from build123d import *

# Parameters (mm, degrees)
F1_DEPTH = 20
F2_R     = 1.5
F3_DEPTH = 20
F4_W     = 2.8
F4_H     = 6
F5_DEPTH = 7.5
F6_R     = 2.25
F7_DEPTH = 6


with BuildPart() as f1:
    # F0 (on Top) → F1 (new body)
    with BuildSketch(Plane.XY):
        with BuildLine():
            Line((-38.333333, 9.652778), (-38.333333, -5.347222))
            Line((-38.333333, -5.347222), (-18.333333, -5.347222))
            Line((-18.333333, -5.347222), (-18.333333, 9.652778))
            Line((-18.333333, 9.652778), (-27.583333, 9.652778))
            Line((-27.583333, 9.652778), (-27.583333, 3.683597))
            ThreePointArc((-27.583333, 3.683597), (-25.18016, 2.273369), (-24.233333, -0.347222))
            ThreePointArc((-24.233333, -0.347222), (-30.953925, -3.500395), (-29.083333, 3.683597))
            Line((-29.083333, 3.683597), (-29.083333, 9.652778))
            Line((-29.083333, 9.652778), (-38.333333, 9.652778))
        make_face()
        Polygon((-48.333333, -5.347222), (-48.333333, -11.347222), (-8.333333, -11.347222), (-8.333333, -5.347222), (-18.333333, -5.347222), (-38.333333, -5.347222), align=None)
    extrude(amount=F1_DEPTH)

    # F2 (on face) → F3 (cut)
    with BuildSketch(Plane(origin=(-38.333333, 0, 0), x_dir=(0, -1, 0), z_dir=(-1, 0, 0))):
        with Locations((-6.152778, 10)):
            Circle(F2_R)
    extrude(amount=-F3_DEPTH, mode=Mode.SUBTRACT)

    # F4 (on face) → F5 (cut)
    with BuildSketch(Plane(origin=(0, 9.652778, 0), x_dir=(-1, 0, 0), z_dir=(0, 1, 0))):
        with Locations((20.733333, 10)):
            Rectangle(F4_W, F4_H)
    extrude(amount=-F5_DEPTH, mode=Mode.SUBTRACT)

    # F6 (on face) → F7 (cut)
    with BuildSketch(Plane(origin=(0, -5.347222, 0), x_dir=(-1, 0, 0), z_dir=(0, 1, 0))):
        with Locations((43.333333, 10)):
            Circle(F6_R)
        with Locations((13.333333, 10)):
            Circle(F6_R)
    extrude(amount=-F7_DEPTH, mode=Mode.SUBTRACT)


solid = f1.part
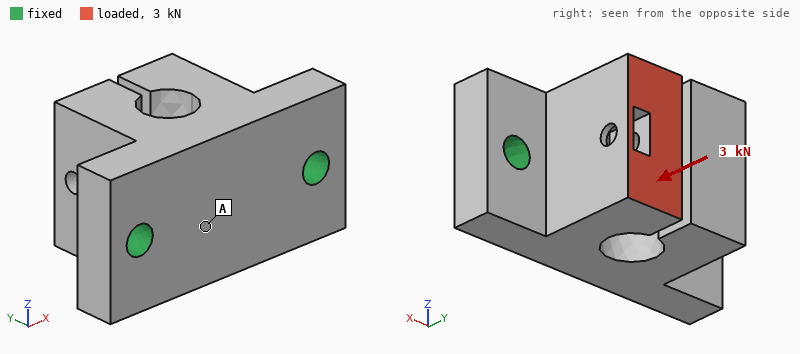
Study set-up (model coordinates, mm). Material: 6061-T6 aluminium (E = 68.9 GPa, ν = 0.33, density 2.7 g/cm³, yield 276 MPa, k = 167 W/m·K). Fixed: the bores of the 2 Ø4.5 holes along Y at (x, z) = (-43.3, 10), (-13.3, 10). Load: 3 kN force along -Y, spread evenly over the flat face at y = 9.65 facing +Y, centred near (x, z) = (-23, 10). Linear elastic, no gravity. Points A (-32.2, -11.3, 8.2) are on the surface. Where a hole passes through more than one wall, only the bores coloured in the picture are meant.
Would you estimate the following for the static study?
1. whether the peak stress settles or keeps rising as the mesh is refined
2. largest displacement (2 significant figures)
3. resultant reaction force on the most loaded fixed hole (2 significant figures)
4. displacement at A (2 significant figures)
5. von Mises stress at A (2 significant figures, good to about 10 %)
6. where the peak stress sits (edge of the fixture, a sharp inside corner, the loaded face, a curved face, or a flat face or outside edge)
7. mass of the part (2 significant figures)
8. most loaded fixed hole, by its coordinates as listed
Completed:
keeps rising
45 µm
2.2 kN
11 µm
15 MPa
edge of the fixture
25 g
(-13.3, 10)
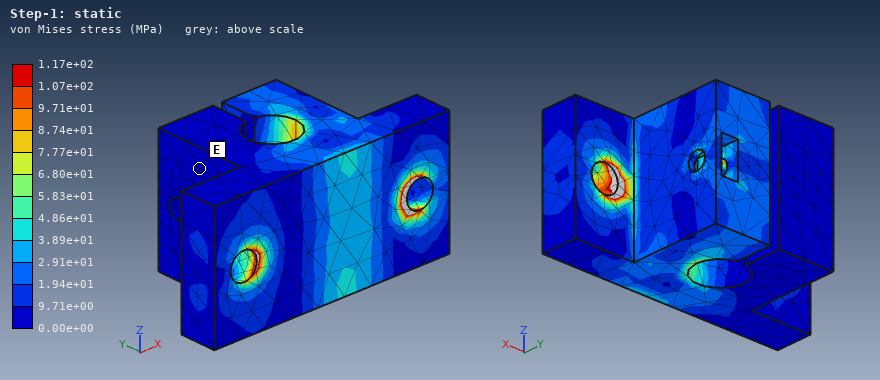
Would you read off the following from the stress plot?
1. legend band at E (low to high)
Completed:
0.00e+00 to 9.71e+00 MPa
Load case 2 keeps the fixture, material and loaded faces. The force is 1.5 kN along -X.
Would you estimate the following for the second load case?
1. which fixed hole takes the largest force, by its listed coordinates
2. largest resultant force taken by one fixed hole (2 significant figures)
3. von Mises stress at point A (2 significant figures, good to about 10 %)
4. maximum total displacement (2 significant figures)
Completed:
(-43.3, 10)
1.4 kN
21 MPa
0.11 mm
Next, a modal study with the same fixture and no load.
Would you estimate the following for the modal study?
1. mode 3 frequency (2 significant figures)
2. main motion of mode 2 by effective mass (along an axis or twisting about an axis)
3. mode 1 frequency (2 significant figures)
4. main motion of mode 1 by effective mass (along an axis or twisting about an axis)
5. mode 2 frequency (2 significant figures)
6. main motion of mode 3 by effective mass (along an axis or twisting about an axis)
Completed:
15 kHz
along Y
9900 Hz
along Z
12 kHz
along X
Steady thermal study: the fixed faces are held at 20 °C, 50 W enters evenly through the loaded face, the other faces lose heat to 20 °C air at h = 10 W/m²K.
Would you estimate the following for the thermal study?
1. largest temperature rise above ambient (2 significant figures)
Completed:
51 K
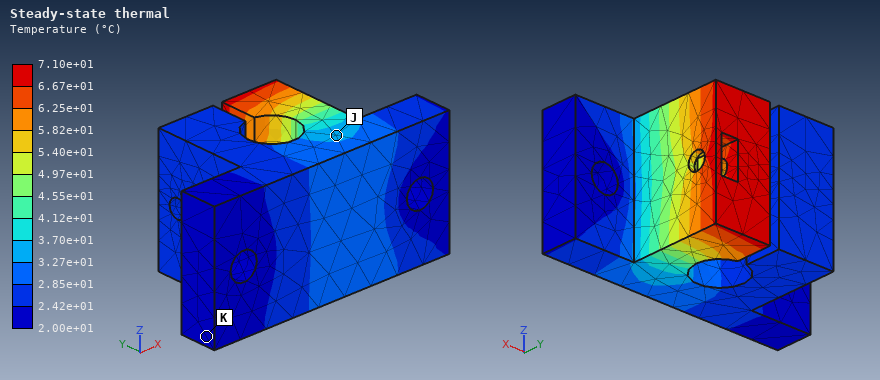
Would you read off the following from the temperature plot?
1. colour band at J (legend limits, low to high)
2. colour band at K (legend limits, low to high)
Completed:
3.27e+01 to 3.70e+01 °C
2.00e+01 to 2.42e+01 °C
